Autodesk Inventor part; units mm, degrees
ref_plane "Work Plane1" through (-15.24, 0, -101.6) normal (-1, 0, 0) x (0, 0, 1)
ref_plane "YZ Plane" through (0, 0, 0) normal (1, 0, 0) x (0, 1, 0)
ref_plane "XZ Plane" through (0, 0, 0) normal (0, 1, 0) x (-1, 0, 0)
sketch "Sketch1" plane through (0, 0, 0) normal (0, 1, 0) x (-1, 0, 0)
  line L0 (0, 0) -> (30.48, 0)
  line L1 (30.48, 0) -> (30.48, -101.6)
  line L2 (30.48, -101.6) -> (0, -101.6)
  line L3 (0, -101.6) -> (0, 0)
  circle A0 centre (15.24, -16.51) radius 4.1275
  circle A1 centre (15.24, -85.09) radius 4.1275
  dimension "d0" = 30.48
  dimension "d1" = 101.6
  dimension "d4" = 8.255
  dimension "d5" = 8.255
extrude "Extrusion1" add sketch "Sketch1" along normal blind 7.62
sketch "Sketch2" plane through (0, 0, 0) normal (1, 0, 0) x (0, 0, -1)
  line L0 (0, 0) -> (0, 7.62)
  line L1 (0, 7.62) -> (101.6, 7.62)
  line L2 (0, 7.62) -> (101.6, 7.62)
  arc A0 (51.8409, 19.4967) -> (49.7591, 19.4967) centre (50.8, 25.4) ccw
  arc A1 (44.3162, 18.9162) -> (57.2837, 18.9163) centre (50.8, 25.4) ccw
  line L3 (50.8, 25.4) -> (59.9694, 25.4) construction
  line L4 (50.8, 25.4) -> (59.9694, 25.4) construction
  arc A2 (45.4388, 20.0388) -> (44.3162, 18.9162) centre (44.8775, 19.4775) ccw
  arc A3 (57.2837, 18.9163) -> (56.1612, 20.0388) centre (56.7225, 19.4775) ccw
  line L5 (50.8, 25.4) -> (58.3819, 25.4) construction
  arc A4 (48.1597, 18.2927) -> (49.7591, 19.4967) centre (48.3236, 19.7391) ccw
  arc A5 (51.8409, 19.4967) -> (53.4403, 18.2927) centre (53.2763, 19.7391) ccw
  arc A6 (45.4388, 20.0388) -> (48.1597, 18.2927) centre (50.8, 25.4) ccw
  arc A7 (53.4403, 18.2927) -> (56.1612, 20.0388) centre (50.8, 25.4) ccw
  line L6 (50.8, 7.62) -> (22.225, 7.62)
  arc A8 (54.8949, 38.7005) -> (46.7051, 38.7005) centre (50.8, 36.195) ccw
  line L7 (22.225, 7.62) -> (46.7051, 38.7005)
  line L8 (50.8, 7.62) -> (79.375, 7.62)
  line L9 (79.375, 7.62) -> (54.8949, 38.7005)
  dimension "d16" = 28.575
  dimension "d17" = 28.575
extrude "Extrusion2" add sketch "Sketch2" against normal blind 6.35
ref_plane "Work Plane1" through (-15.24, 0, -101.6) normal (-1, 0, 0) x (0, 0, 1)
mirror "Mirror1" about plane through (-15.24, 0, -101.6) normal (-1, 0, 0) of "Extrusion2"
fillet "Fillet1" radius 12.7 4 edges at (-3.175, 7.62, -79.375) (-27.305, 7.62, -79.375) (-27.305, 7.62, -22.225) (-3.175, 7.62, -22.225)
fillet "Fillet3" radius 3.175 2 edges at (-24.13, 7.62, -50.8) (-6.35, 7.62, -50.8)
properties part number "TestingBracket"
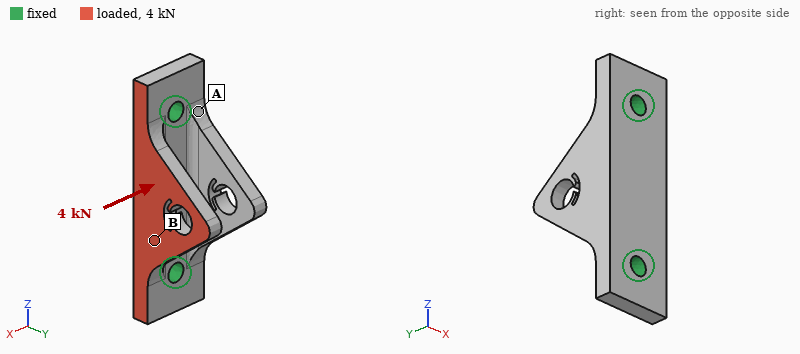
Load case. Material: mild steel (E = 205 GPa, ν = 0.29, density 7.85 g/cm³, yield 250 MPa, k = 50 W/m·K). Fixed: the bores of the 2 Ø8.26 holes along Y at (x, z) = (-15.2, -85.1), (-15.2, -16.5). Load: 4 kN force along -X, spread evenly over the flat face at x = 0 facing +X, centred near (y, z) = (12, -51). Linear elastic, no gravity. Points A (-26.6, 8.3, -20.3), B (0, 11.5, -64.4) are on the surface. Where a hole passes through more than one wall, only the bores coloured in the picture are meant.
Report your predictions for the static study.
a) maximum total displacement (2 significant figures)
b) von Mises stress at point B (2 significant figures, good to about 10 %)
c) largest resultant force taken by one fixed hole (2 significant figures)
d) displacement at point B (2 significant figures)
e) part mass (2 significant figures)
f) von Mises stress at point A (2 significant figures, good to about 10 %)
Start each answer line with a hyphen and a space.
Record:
- 85 µm
- 53 MPa
- 2.0 kN
- 17 µm
- 270 g
- 13 MPa
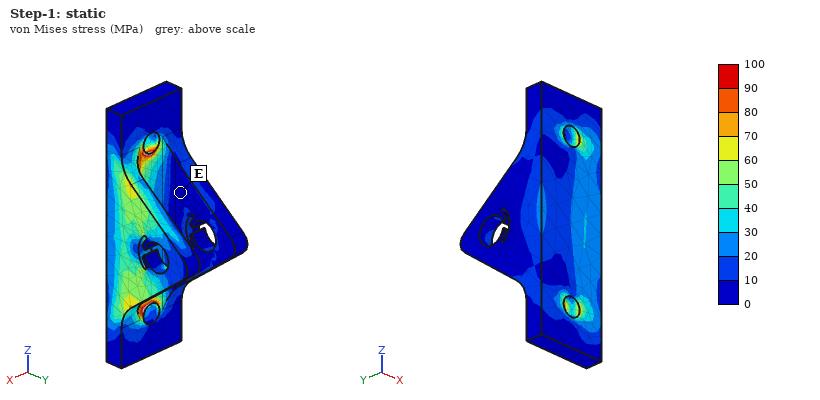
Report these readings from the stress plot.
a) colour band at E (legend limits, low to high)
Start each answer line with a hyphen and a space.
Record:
- 0 to 10 MPa
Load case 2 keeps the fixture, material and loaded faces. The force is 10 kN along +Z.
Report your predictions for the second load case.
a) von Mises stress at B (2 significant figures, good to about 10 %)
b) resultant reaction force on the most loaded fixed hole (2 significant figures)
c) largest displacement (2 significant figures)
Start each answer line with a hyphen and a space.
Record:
- 25 MPa
- 5.5 kN
- 16 µm
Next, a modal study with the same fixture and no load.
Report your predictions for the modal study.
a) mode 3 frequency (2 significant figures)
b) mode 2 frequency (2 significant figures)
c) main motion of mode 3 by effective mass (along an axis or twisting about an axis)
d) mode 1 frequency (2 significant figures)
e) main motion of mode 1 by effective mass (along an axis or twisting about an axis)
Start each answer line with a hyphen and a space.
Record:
- 9500 Hz
- 5800 Hz
- along Y
- 4600 Hz
- along X
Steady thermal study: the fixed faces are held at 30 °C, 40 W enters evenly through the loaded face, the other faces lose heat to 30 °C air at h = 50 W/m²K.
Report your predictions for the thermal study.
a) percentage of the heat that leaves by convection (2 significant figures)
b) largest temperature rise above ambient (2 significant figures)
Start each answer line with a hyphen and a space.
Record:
- 19 %
- 49 K
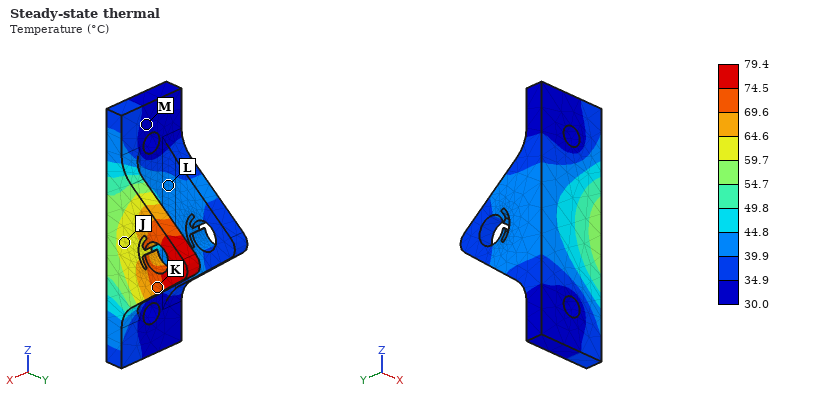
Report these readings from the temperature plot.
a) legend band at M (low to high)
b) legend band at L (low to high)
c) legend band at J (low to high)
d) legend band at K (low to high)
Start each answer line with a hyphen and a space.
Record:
- 30.0 to 34.9 °C
- 39.9 to 44.8 °C
- 59.7 to 64.6 °C
- 69.6 to 74.5 °C
